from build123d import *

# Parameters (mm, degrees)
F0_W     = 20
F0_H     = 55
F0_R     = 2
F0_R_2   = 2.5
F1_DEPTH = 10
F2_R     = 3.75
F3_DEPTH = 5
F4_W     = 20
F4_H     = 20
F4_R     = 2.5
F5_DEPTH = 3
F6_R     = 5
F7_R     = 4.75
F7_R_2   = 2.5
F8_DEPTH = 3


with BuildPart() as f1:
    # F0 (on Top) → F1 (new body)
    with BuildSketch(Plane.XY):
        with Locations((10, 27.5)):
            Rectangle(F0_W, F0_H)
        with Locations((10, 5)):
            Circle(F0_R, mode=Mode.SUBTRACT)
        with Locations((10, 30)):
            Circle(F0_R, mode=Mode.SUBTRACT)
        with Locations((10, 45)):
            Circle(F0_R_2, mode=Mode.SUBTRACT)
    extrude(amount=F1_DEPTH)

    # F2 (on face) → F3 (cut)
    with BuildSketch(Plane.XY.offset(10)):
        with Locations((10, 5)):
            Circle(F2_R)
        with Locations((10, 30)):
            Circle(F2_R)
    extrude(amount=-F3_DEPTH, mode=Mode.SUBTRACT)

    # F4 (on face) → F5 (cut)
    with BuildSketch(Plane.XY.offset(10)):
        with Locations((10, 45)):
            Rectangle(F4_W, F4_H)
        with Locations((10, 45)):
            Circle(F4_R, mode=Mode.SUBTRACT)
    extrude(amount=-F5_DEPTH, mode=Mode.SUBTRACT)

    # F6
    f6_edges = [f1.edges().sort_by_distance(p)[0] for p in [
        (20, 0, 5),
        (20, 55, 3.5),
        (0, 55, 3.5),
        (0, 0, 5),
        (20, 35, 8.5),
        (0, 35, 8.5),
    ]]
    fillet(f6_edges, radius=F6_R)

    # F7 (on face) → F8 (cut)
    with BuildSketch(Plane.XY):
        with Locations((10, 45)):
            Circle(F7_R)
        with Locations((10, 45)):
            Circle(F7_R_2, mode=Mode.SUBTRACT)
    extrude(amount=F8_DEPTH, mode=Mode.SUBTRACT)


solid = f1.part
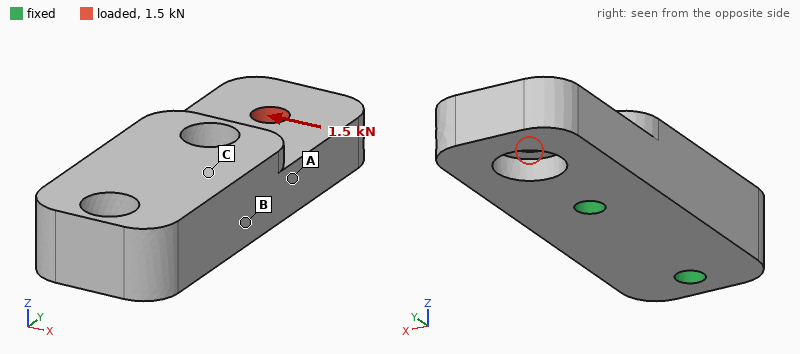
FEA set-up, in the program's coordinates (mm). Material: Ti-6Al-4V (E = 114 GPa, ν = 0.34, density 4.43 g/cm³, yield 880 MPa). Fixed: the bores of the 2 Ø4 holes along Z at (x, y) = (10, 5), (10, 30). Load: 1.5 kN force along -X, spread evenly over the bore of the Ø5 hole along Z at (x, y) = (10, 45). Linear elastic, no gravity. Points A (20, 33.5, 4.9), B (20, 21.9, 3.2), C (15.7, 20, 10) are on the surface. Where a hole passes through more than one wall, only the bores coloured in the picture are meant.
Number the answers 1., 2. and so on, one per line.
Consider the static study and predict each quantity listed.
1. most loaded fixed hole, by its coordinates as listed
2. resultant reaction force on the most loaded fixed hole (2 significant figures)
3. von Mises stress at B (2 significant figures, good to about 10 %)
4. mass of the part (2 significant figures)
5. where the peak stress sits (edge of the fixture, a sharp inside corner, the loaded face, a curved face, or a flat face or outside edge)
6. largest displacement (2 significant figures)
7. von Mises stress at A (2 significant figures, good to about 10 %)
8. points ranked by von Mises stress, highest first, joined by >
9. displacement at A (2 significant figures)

1. (10, 30)
2. 2.2 kN
3. 22 MPa
4. 39 g
5. edge of the fixture
6. 25 µm
7. 42 MPa
8. A > B > C
9. 7.7 µm
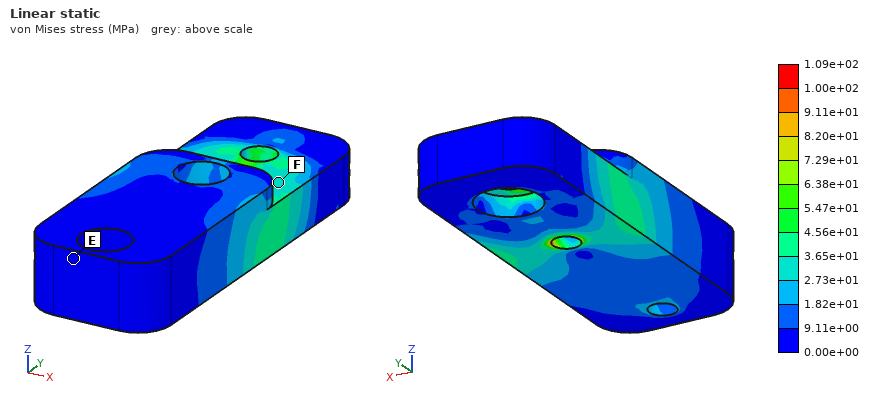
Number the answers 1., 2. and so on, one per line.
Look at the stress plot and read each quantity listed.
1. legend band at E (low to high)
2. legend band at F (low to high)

1. 0.00e+00 to 9.11e+00 MPa
2. 2.73e+01 to 3.65e+01 MPa
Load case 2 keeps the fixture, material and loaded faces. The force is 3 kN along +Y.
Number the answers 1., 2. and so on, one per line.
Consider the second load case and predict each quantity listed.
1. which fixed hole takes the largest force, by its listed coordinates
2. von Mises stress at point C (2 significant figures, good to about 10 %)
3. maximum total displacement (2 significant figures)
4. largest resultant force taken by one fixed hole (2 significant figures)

1. (10, 30)
2. 9.2 MPa
3. 22 µm
4. 2.3 kN
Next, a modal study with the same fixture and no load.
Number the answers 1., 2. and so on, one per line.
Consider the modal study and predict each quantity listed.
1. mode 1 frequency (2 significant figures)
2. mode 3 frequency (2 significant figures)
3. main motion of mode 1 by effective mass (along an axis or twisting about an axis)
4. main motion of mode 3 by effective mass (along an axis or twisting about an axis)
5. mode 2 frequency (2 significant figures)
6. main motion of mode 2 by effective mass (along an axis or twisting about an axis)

1. 8600 Hz
2. 15 kHz
3. along Z
4. twisting about Y
5. 14 kHz
6. along X
